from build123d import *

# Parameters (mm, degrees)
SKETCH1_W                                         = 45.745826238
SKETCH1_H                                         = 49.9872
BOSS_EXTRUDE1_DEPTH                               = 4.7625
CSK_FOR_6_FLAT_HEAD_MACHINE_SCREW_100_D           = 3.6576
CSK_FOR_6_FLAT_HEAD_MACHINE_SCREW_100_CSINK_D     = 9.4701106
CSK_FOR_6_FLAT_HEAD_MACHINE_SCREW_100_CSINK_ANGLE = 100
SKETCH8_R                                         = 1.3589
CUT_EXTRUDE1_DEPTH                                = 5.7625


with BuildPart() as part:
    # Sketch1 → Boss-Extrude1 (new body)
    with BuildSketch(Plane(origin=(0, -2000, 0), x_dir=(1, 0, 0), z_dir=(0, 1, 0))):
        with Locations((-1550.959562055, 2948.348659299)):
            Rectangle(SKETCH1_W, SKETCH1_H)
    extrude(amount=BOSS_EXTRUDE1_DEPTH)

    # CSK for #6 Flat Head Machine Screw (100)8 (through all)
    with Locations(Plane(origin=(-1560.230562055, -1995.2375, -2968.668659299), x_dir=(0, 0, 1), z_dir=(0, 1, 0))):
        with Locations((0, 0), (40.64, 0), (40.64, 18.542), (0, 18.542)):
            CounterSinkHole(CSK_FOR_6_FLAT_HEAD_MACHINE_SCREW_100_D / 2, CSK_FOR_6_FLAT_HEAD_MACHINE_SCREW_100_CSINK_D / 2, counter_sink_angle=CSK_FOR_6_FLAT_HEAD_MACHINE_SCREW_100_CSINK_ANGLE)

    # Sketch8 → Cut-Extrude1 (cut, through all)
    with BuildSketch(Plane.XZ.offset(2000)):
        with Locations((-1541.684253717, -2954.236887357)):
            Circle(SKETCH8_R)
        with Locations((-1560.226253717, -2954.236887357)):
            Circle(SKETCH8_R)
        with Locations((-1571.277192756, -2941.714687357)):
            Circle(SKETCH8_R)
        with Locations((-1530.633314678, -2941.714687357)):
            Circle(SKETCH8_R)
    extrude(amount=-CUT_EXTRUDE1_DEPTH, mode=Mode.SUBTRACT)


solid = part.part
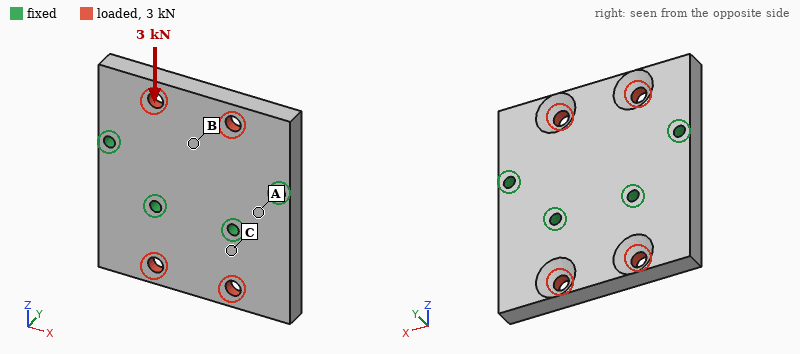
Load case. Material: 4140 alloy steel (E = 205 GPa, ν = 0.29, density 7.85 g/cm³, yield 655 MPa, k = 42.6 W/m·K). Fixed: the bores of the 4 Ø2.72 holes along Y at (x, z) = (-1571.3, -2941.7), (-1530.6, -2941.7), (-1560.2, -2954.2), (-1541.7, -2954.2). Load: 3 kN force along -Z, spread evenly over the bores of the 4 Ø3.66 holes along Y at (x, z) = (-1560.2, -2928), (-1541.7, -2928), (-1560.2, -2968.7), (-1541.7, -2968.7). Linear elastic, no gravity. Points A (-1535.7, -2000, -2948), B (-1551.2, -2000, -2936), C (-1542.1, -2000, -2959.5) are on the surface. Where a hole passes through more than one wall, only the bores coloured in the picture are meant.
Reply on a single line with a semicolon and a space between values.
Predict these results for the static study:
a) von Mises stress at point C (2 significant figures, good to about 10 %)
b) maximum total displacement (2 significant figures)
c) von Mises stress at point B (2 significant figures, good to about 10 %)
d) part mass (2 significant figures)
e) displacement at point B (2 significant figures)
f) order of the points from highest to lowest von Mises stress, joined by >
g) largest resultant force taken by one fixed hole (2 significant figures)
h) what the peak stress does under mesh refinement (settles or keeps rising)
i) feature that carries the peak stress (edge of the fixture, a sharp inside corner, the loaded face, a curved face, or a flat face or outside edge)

27 MPa; 6.2 µm; 14 MPa; 81 g; 2.2 µm; C > B > A; 980 N; keeps rising; edge of the fixture
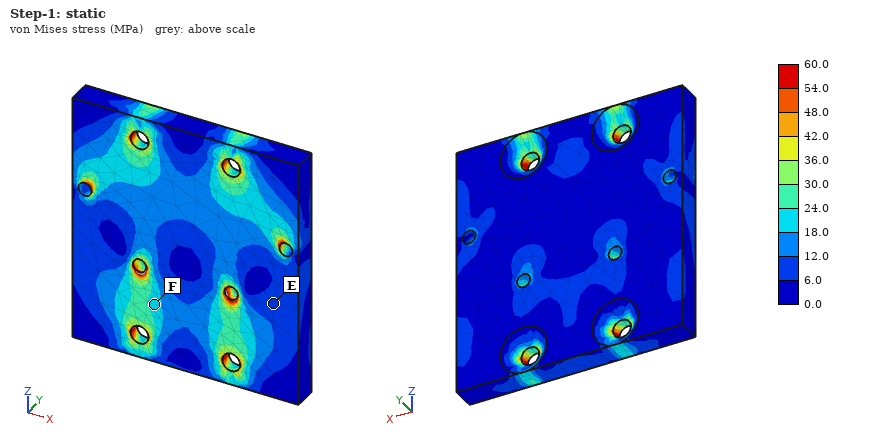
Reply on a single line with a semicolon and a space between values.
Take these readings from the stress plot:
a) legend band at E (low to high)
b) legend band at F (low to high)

6.0 to 12.0 MPa; 18.0 to 24.0 MPa
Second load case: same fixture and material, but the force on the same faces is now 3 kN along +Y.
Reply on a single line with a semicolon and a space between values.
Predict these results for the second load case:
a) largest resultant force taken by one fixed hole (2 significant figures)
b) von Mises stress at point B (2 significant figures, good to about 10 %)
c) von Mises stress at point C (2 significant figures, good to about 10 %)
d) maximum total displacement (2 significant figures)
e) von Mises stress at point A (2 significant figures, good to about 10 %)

910 N; 60 MPa; 91 MPa; 57 µm; 52 MPa
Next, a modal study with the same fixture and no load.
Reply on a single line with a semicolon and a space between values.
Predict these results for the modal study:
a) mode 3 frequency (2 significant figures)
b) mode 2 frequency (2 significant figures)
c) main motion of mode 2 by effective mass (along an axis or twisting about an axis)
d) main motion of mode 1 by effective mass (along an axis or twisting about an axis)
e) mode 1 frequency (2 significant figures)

11 kHz; 9300 Hz; along Y; along Y; 7800 Hz
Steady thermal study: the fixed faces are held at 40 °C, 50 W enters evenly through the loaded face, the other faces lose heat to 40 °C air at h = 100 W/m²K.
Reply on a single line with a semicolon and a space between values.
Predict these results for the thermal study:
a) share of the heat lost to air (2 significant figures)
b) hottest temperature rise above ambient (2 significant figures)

27 %; 66 K
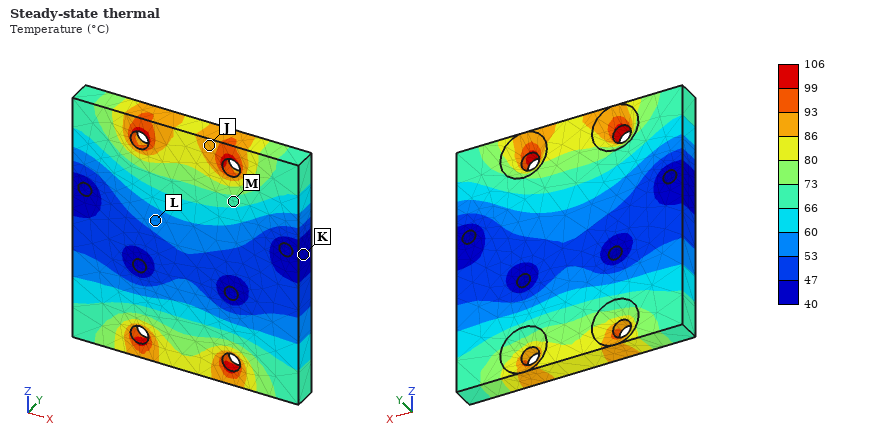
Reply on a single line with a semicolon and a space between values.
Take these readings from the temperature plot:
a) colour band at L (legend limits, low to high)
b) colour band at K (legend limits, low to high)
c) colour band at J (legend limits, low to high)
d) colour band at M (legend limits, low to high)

53 to 60 °C; 40 to 47 °C; 86 to 93 °C; 66 to 73 °C
